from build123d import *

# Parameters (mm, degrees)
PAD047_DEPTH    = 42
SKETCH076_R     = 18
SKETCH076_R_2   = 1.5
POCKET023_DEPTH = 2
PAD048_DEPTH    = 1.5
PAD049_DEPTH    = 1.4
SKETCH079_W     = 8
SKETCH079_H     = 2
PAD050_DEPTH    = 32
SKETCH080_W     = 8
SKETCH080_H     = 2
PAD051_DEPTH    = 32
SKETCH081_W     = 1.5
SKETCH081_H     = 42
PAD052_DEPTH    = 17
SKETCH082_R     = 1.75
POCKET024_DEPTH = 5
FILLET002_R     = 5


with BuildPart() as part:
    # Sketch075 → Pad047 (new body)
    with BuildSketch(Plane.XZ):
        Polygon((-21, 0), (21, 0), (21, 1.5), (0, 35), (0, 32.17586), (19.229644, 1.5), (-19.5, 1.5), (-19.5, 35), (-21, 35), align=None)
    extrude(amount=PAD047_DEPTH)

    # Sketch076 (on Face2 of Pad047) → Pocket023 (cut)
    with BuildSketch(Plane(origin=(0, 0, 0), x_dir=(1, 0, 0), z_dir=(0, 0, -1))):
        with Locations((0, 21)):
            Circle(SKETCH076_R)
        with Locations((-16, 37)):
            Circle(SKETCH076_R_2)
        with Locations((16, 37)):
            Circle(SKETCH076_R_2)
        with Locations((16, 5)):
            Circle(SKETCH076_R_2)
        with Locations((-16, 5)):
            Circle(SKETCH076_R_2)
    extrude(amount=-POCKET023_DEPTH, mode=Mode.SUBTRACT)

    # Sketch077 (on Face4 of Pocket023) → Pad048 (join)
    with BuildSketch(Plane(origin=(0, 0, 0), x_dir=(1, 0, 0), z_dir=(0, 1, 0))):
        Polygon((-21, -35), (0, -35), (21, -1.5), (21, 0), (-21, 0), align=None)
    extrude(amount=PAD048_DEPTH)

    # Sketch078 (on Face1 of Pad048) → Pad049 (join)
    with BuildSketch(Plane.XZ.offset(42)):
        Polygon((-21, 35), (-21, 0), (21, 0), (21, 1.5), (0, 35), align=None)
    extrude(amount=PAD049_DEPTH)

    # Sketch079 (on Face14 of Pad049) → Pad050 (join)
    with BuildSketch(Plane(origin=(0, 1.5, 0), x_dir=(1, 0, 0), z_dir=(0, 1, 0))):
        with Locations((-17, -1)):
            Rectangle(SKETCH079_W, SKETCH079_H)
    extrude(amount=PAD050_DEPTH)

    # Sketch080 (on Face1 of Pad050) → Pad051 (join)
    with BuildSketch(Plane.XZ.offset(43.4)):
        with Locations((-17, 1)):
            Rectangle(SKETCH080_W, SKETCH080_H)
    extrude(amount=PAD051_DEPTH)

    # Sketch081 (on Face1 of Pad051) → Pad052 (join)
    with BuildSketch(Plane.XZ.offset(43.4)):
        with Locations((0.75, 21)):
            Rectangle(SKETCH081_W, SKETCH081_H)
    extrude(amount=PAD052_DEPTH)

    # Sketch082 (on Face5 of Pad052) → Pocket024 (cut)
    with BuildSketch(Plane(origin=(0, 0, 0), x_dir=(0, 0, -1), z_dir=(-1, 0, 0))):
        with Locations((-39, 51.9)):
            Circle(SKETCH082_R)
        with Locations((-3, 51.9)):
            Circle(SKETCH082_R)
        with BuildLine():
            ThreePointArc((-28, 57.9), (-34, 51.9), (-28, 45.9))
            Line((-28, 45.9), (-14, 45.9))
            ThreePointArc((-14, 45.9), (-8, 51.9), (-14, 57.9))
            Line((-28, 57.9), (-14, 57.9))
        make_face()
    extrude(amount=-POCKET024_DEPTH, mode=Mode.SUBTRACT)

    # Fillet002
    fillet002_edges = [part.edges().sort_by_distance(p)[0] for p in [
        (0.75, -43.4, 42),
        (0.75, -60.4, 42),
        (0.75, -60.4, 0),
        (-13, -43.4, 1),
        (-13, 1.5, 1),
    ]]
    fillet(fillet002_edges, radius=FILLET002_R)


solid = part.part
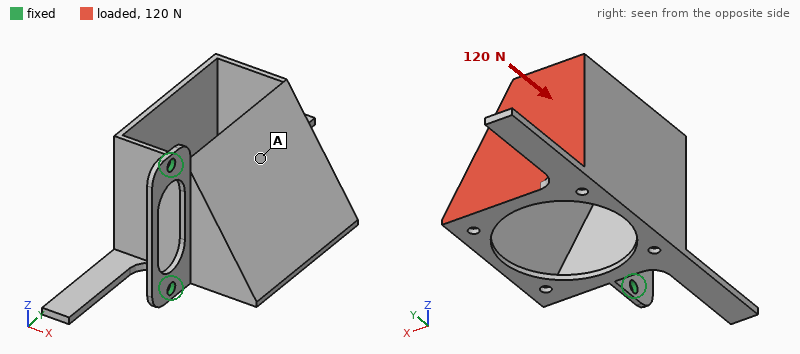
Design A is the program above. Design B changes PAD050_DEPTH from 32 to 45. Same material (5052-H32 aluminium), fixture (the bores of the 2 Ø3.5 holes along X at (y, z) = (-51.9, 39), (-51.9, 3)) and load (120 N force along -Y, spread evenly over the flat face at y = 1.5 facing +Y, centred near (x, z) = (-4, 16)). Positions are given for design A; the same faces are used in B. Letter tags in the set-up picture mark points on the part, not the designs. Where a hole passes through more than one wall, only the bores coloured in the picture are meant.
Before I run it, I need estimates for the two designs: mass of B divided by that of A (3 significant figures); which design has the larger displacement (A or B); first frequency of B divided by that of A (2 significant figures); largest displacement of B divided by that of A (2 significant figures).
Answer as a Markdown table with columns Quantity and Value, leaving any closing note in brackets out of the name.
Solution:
| Quantity | Value |
|---|---|
| mass of B divided by that of A | 1.02 |
| which design has the larger displacement | B |
| first frequency of B divided by that of A | 0.94 |
| largest displacement of B divided by that of A | 1.2 |
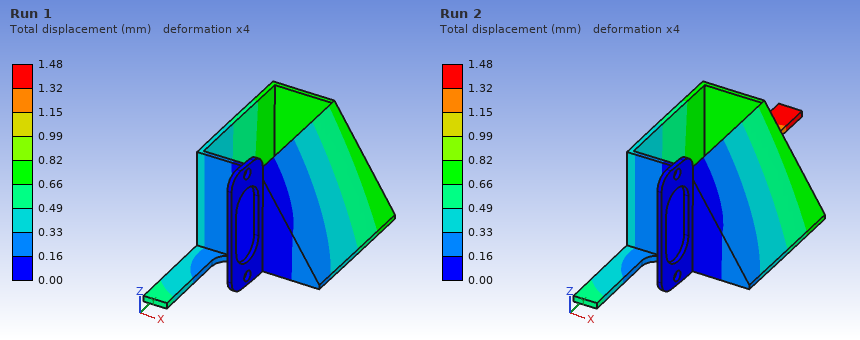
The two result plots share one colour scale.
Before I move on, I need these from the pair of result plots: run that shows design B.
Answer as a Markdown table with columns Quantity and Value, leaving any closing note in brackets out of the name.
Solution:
| Quantity | Value |
|---|---|
| run that shows design B | Run 2 |
